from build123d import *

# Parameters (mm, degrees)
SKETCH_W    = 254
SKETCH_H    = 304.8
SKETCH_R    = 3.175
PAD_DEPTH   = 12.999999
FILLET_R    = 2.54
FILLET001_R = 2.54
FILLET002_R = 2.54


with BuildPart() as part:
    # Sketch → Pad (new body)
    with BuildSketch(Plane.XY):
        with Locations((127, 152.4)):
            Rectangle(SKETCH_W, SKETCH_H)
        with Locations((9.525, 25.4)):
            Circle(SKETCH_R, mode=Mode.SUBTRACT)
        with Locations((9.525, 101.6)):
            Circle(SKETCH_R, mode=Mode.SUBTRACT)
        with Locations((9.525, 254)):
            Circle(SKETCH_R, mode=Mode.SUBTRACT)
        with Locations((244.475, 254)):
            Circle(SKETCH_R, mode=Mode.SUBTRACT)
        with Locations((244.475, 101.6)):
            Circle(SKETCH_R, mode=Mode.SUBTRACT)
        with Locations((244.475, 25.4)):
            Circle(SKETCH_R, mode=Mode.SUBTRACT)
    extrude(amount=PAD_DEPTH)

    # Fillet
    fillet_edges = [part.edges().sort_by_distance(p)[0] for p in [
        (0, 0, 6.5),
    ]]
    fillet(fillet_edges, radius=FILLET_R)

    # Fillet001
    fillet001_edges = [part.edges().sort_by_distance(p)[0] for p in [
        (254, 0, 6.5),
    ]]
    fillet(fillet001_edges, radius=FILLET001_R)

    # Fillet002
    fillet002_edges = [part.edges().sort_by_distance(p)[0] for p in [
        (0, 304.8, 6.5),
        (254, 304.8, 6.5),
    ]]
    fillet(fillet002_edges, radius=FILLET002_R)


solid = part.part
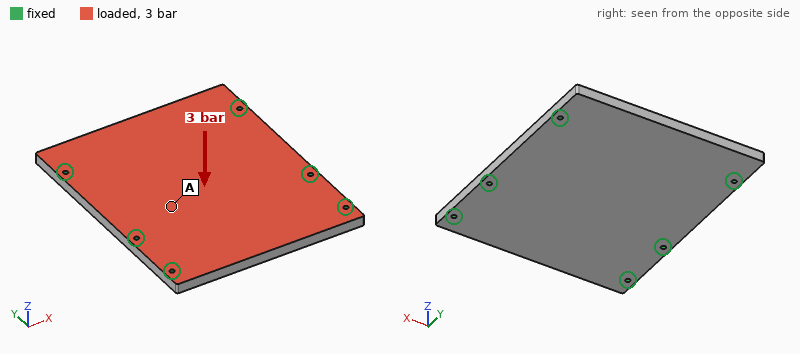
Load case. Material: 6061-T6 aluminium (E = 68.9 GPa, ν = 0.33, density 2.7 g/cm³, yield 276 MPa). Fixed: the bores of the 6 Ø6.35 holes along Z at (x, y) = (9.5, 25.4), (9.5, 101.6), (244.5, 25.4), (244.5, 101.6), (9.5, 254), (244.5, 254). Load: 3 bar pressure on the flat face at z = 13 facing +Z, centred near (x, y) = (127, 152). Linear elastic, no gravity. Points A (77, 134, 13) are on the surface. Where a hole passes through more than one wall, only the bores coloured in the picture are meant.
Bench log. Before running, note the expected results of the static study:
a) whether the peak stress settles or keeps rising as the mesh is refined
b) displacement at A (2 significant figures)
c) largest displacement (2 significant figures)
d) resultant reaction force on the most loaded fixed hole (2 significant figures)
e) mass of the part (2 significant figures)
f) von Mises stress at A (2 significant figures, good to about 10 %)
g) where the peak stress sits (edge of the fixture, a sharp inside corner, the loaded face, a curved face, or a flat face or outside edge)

keeps rising
0.25 mm
0.38 mm
4.9 kN
2.7 kg
19 MPa
edge of the fixture
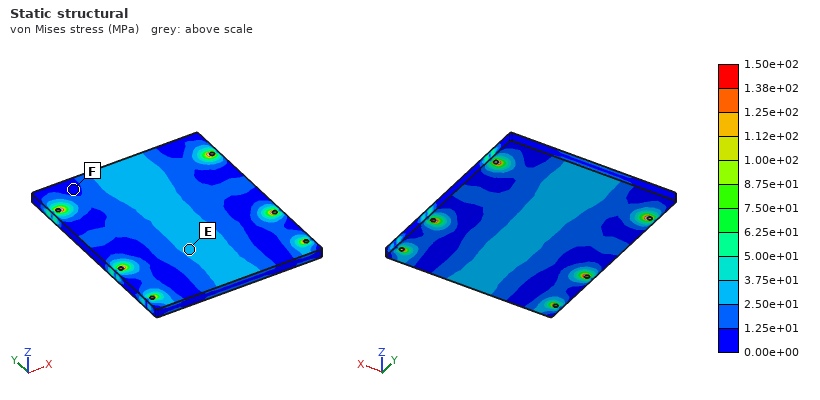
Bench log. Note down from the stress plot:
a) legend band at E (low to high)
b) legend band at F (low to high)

2.50e+01 to 3.75e+01 MPa
0.00e+00 to 1.25e+01 MPa
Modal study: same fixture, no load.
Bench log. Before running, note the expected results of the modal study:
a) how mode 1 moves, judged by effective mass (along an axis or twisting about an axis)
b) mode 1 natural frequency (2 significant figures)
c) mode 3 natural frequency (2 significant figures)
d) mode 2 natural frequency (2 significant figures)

along Z
910 Hz
1500 Hz
1100 Hz
